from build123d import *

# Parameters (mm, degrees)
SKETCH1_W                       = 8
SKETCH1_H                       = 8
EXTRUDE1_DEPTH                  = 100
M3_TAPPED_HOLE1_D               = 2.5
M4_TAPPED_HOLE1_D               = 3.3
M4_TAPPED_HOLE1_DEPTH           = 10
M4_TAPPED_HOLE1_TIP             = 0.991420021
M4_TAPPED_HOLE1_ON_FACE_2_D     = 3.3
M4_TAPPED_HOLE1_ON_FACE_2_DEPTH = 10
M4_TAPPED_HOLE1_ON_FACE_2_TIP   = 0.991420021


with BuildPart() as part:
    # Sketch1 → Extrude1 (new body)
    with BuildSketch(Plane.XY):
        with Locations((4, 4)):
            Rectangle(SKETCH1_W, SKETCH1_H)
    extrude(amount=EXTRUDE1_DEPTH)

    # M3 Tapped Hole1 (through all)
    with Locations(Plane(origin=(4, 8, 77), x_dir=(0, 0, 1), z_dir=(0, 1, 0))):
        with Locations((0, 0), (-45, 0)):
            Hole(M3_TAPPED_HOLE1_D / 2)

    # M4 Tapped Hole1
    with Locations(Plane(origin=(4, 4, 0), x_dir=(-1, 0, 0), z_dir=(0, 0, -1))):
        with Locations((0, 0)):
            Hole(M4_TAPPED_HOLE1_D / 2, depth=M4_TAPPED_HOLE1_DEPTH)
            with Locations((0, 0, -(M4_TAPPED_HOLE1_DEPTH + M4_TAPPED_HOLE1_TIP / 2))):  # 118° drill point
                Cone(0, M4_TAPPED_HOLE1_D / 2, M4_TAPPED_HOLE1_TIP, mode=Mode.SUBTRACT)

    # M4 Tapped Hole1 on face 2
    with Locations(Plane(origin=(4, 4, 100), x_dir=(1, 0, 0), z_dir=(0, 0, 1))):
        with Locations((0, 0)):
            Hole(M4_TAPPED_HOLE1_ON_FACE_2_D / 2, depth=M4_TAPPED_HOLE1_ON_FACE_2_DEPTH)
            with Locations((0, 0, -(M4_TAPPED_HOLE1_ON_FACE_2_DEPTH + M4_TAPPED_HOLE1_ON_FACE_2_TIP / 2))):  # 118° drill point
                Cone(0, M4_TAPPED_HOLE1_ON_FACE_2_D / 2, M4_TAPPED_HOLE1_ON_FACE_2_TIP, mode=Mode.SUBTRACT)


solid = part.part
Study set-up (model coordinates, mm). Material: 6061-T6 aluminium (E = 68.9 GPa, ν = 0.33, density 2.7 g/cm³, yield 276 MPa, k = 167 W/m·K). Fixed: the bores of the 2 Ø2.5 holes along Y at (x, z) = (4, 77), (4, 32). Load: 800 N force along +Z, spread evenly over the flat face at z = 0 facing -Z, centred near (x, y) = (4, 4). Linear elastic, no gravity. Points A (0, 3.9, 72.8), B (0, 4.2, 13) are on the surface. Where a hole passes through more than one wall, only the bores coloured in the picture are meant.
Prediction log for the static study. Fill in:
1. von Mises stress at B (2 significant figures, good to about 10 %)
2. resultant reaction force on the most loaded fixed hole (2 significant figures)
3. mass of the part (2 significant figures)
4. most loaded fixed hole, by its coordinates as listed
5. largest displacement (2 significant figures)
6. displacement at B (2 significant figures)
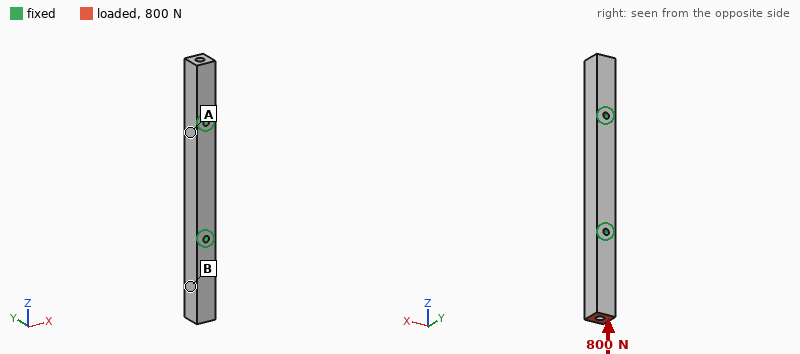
13 MPa
780 N
17 g
(4, 32)
6.2 µm
3.5 µm
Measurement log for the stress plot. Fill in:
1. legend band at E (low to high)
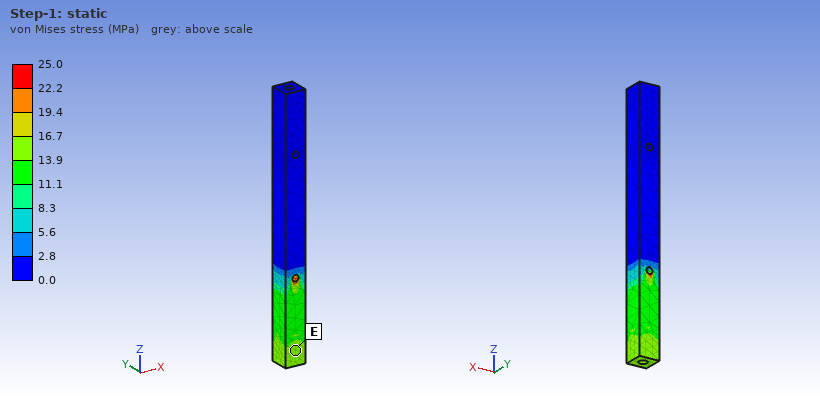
13.9 to 16.7 MPa
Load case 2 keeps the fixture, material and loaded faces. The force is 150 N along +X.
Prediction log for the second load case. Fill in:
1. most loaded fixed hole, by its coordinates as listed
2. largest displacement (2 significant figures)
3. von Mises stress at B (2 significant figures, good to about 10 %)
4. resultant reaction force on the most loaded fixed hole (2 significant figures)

(4, 32)
96 µm
23 MPa
190 N
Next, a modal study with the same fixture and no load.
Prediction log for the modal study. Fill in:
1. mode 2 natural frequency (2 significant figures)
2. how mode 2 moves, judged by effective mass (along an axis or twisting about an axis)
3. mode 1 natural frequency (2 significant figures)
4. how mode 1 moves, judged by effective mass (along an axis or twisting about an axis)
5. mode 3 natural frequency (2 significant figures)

6400 Hz
along Y
5500 Hz
along X
9700 Hz
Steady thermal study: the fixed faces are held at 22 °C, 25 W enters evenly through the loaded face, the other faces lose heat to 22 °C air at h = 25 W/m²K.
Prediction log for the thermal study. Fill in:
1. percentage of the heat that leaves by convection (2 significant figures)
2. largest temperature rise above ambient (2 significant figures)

4.4 %
76 K
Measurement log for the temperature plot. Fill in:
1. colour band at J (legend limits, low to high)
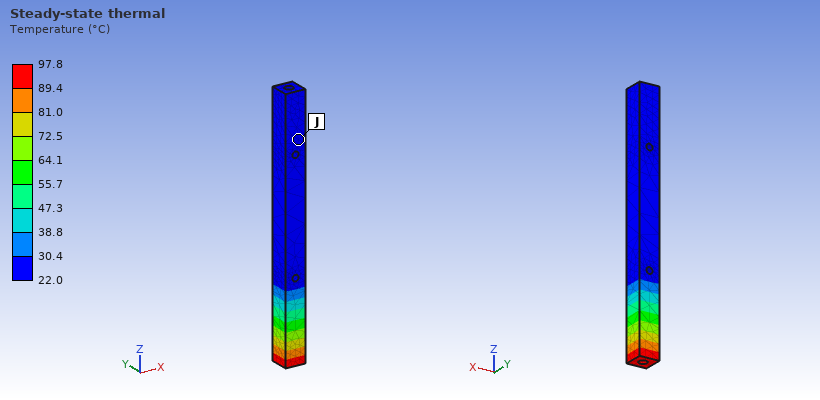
22.0 to 30.4 °C
